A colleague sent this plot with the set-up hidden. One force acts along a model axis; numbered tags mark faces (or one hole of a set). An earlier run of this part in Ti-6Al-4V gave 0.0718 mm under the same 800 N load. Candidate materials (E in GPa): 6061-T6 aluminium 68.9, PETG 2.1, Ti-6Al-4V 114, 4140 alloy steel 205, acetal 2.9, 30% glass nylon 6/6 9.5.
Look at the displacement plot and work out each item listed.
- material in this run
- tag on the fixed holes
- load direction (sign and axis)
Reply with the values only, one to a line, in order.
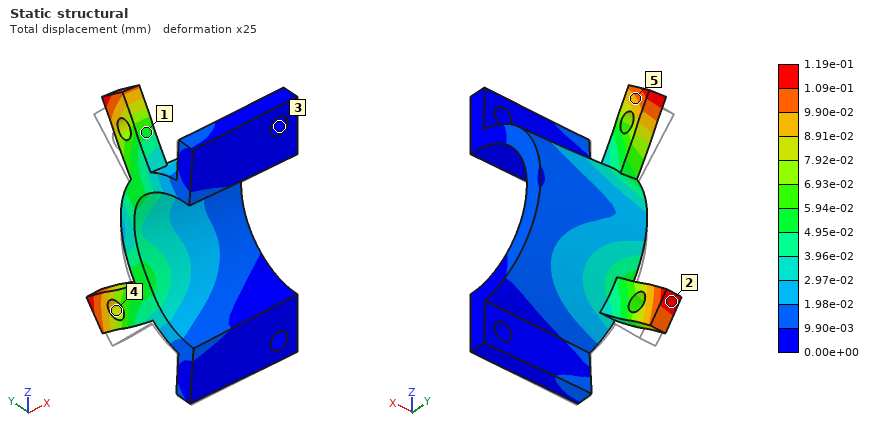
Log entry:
6061-T6 aluminium
3
+Z
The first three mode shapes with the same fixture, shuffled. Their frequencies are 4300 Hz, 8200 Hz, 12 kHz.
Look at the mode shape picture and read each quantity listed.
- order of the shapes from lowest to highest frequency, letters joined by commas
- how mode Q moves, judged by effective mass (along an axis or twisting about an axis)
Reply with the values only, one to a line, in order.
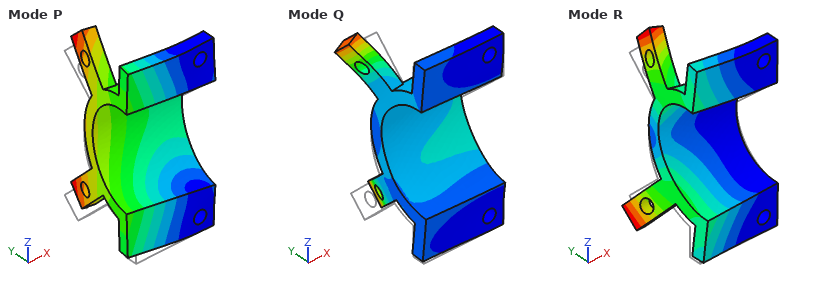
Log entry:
P, R, Q
along Z
